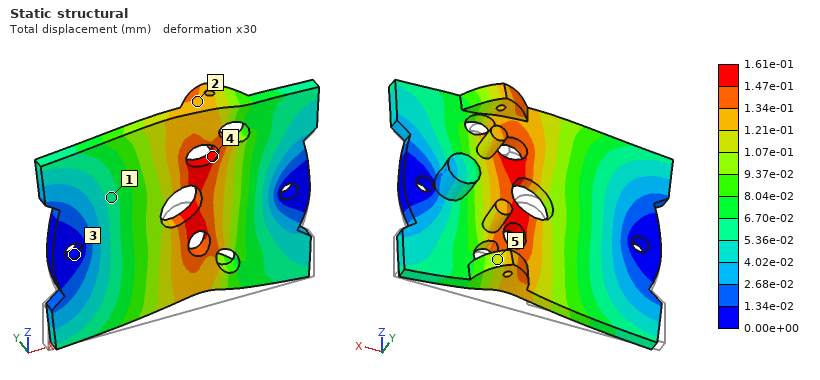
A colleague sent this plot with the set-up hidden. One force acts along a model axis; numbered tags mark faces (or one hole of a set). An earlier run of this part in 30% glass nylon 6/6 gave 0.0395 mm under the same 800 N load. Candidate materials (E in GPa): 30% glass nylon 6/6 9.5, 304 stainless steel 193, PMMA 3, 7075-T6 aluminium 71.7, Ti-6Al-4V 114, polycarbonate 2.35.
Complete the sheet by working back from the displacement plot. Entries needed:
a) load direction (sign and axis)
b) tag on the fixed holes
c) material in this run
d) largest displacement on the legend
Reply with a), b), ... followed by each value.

a) +Z
b) 3
c) polycarbonate
d) 1.61e-01 mm
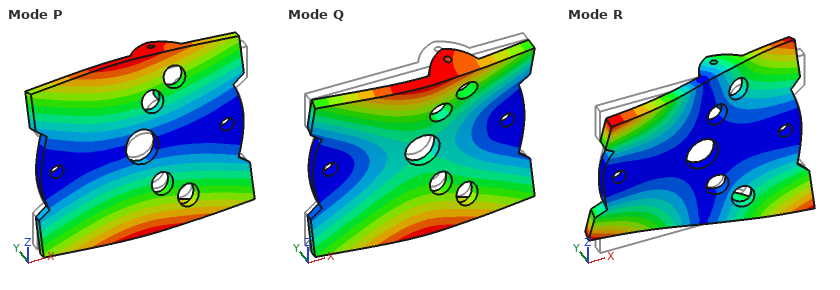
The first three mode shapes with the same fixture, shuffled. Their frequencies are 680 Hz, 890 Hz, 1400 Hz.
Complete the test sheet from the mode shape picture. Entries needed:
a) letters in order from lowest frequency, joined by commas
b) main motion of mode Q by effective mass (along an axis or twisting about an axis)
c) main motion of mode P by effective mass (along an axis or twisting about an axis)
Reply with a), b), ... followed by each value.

a) P, Q, R
b) along Y
c) twisting about X
